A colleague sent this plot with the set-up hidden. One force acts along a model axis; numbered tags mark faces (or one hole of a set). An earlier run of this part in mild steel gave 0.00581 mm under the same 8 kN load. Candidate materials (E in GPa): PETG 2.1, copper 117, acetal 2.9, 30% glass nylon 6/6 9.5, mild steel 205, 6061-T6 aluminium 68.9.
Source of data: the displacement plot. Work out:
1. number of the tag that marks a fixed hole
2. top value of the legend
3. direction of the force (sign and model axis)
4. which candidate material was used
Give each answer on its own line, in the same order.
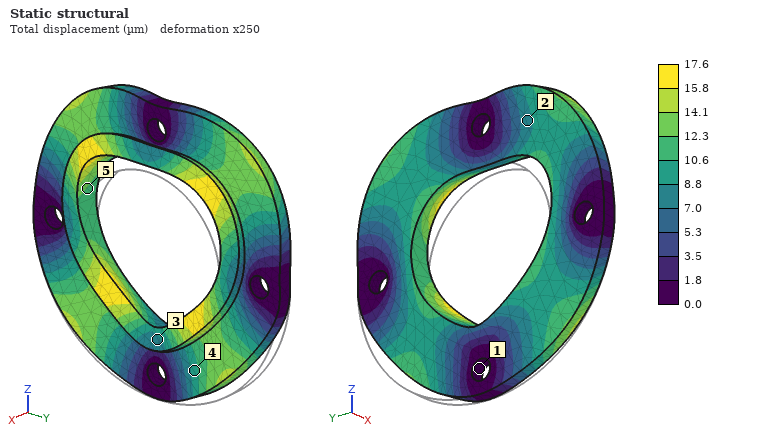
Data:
1
17.6 µm
+Z
6061-T6 aluminium
